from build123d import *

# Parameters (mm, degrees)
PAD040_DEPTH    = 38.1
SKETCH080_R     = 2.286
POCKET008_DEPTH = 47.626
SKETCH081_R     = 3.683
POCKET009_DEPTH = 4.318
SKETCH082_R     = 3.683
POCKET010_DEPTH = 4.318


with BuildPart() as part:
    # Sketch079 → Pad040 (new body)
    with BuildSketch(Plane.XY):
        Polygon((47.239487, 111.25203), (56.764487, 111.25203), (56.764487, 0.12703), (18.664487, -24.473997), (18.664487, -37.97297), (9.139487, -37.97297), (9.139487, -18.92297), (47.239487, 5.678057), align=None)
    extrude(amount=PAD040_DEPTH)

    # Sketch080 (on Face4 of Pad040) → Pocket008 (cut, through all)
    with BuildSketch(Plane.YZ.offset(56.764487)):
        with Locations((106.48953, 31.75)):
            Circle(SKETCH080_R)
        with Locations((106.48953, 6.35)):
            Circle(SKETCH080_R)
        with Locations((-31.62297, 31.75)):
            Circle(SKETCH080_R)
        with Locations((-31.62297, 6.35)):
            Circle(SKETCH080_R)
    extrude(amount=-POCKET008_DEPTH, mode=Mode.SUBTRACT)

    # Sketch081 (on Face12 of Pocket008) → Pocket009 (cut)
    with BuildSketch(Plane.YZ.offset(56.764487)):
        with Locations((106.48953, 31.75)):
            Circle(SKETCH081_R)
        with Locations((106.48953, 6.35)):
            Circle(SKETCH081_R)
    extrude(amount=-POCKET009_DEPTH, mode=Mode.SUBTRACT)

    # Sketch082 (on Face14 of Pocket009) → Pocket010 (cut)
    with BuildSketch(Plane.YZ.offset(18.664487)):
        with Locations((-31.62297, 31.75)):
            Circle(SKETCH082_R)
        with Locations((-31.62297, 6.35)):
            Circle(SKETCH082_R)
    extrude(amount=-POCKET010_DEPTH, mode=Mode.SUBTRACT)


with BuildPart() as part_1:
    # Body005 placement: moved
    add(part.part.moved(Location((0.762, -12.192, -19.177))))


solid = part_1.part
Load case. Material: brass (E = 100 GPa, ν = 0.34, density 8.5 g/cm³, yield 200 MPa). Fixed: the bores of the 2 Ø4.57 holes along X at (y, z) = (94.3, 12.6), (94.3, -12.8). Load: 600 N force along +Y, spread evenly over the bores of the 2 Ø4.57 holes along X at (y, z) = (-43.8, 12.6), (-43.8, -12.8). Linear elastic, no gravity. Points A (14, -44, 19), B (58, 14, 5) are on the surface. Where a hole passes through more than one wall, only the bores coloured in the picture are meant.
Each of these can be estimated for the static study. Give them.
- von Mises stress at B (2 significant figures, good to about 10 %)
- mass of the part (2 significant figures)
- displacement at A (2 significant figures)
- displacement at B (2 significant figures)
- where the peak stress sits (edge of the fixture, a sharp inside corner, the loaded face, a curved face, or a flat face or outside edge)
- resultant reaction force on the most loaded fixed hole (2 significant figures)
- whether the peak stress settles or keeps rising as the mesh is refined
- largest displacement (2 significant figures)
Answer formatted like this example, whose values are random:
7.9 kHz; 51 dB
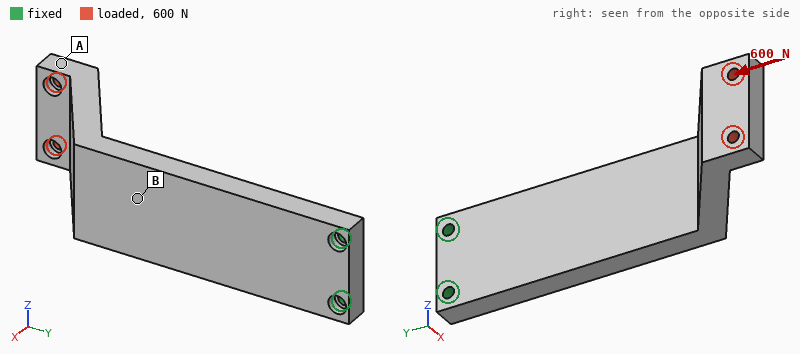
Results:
39 MPa; 520 g; 1.1 mm; 0.38 mm; edge of the fixture; 330 N; keeps rising; 1.2 mm
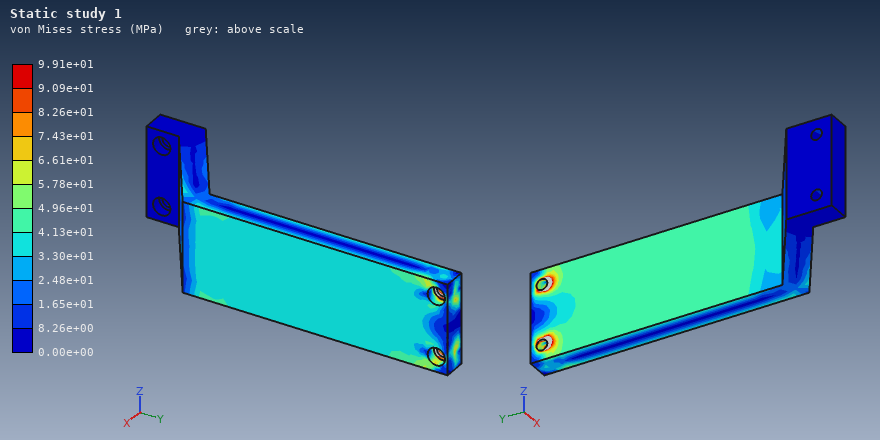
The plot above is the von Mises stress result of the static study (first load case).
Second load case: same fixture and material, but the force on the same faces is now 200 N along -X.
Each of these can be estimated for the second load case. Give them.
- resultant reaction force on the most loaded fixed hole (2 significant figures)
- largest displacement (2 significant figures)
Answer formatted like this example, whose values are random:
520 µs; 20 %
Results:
130 N; 0.96 mm
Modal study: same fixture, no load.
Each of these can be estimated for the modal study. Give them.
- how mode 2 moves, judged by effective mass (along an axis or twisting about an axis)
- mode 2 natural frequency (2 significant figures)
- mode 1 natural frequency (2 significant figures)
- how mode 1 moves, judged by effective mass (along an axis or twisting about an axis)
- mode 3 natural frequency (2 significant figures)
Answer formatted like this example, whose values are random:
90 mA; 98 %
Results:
along Z; 560 Hz; 180 Hz; along X; 970 Hz
